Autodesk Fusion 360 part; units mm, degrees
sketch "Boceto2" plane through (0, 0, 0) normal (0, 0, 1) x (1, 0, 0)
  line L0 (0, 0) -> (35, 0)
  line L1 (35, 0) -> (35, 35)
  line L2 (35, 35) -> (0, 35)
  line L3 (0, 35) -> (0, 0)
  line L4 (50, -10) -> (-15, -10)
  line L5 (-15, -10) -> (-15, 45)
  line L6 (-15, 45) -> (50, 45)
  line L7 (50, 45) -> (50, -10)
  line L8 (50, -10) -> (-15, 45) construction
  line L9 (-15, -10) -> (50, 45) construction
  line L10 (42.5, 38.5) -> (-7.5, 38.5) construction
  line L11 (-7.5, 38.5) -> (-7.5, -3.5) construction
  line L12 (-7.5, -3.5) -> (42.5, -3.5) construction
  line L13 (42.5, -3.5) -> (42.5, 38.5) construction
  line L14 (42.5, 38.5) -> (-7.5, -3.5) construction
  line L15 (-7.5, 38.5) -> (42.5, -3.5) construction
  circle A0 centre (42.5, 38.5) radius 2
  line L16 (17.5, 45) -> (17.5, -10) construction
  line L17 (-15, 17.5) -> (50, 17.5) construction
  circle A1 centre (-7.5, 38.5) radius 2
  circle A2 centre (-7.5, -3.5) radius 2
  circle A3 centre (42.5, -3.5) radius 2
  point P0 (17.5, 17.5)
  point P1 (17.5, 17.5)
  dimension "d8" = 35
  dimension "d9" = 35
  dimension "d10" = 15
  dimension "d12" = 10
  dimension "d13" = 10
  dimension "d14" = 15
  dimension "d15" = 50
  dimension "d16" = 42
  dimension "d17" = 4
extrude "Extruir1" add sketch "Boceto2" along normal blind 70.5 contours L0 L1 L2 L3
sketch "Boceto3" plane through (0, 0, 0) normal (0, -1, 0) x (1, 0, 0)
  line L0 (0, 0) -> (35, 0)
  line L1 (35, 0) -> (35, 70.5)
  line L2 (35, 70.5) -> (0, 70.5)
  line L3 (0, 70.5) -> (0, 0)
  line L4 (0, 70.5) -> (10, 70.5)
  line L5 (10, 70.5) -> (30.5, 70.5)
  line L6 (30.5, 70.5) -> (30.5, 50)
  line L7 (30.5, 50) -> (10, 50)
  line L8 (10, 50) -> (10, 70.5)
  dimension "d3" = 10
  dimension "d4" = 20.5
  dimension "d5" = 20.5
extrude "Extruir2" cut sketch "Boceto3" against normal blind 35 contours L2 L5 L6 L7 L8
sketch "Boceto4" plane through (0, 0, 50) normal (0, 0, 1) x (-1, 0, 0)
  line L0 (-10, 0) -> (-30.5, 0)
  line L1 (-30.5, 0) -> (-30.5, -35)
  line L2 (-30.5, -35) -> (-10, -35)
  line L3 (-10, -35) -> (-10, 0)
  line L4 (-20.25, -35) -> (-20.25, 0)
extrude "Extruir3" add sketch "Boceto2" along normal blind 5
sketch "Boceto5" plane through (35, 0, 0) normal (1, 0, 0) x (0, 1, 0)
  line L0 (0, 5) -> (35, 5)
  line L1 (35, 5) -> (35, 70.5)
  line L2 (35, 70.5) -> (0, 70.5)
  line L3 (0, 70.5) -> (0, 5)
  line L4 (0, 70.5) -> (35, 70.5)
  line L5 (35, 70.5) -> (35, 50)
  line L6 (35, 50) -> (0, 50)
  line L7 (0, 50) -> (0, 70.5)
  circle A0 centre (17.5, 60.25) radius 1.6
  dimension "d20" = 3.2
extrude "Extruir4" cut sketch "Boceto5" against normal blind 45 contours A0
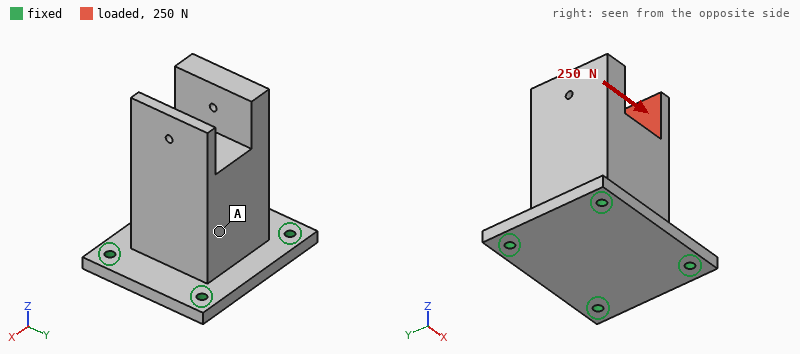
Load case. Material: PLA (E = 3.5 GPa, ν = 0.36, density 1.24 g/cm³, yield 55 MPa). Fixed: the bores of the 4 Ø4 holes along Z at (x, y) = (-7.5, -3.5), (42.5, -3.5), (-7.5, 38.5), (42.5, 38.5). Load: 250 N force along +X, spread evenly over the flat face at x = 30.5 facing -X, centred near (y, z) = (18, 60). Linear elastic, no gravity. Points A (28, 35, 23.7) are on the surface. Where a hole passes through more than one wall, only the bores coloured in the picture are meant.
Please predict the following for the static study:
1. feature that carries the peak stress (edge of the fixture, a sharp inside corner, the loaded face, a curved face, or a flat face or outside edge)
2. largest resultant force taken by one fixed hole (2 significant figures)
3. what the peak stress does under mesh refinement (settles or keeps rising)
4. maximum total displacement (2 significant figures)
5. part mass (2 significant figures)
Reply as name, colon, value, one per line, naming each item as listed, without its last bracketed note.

feature that carries the peak stress: edge of the fixture
largest resultant force taken by one fixed hole: 180 N
what the peak stress does under mesh refinement: keeps rising
maximum total displacement: 0.71 mm
part mass: 100 g
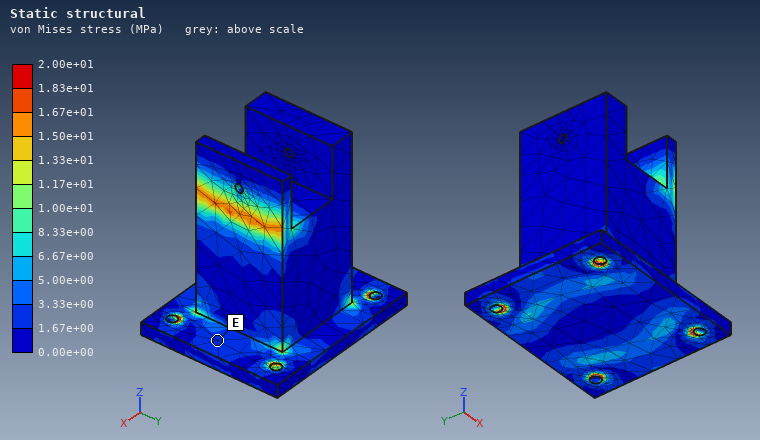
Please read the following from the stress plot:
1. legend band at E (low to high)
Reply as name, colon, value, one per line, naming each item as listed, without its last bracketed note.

legend band at E: 1.67e+00 to 3.33e+00 MPa
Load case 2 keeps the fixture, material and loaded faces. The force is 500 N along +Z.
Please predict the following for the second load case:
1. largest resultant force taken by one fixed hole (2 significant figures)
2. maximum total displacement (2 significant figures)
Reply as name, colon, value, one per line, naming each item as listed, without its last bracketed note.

largest resultant force taken by one fixed hole: 210 N
maximum total displacement: 0.15 mm
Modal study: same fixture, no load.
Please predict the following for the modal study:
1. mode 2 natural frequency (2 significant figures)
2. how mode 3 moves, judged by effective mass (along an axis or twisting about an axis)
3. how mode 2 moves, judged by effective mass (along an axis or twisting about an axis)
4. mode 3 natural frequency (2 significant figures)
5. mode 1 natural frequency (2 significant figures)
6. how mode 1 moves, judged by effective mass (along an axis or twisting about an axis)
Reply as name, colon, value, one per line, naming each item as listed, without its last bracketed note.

mode 2 natural frequency: 950 Hz
how mode 3 moves, judged by effective mass: along Z
how mode 2 moves, judged by effective mass: along X
mode 3 natural frequency: 1600 Hz
mode 1 natural frequency: 850 Hz
how mode 1 moves, judged by effective mass: along Y
